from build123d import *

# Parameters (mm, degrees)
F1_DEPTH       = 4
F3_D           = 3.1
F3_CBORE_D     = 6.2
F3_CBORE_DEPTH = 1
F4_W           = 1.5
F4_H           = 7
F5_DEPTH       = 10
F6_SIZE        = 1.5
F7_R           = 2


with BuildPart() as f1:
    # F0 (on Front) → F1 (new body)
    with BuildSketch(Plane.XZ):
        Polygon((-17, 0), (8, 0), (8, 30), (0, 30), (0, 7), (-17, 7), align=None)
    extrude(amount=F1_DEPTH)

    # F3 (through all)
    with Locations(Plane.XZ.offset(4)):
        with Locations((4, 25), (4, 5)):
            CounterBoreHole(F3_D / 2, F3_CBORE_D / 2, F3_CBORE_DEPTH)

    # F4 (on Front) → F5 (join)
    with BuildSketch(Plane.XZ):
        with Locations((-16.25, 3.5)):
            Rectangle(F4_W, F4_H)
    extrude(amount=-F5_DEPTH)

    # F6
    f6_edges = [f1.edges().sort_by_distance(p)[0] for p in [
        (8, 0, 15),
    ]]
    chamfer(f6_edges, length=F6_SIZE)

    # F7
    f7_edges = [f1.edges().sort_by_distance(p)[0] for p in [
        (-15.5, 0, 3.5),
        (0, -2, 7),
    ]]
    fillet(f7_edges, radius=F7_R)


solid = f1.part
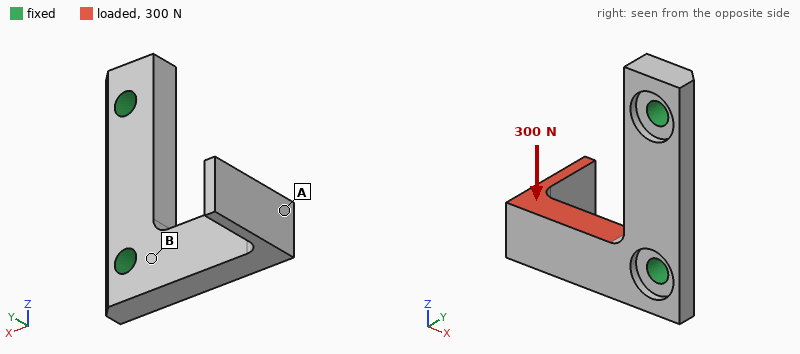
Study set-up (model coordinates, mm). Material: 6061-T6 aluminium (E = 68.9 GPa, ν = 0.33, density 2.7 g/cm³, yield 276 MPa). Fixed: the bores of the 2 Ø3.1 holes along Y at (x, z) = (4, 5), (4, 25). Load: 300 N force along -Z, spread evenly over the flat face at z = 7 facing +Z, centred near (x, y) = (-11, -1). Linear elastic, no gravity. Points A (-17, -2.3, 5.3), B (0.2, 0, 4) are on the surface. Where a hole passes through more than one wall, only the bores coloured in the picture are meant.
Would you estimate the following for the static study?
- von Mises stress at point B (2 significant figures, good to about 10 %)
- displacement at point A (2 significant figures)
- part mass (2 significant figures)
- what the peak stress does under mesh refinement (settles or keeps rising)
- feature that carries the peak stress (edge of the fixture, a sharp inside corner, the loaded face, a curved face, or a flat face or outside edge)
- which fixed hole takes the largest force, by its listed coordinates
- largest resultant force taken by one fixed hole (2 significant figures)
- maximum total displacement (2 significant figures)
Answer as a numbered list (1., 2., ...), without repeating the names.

1. 43 MPa
2. 0.075 mm
3. 3.8 g
4. keeps rising
5. edge of the fixture
6. (4, 5)
7. 220 N
8. 0.12 mm
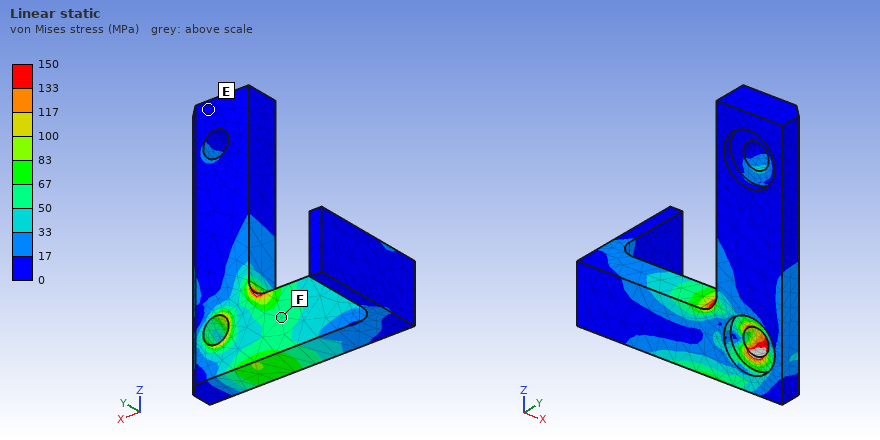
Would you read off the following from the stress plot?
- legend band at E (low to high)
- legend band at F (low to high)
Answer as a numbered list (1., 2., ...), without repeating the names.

1. 0 to 17 MPa
2. 50 to 67 MPa
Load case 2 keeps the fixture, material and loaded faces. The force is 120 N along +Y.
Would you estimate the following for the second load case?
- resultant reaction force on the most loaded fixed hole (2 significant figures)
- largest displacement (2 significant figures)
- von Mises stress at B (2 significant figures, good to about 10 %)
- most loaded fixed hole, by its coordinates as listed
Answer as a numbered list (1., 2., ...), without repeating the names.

1. 130 N
2. 0.13 mm
3. 78 MPa
4. (4, 5)
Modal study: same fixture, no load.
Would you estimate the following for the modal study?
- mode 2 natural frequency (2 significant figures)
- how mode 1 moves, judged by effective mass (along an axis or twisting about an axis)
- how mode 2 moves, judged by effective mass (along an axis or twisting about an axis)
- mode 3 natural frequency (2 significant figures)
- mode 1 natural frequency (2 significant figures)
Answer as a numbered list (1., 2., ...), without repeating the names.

1. 8400 Hz
2. along Y
3. along Z
4. 12 kHz
5. 5100 Hz
